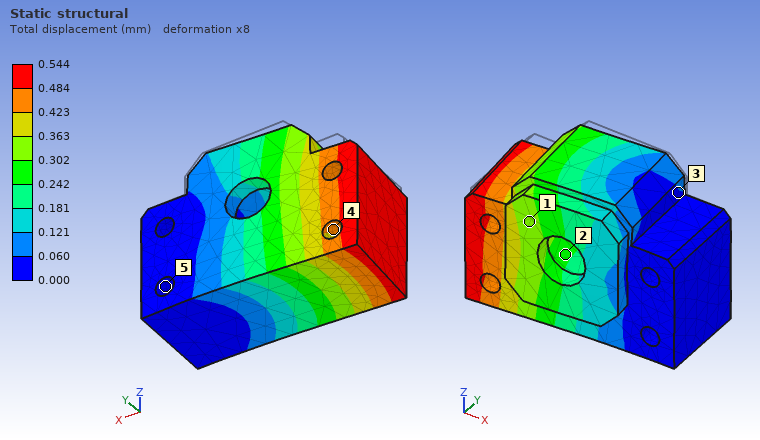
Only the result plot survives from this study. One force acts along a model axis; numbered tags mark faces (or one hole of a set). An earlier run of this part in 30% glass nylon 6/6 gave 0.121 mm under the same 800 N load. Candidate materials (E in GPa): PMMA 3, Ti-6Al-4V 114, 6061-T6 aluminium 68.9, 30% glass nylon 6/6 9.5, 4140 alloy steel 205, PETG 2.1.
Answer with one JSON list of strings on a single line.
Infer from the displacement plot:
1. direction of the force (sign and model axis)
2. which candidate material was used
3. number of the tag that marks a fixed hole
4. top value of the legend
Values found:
["-Y", "PETG", "5", "0.544 mm"]
